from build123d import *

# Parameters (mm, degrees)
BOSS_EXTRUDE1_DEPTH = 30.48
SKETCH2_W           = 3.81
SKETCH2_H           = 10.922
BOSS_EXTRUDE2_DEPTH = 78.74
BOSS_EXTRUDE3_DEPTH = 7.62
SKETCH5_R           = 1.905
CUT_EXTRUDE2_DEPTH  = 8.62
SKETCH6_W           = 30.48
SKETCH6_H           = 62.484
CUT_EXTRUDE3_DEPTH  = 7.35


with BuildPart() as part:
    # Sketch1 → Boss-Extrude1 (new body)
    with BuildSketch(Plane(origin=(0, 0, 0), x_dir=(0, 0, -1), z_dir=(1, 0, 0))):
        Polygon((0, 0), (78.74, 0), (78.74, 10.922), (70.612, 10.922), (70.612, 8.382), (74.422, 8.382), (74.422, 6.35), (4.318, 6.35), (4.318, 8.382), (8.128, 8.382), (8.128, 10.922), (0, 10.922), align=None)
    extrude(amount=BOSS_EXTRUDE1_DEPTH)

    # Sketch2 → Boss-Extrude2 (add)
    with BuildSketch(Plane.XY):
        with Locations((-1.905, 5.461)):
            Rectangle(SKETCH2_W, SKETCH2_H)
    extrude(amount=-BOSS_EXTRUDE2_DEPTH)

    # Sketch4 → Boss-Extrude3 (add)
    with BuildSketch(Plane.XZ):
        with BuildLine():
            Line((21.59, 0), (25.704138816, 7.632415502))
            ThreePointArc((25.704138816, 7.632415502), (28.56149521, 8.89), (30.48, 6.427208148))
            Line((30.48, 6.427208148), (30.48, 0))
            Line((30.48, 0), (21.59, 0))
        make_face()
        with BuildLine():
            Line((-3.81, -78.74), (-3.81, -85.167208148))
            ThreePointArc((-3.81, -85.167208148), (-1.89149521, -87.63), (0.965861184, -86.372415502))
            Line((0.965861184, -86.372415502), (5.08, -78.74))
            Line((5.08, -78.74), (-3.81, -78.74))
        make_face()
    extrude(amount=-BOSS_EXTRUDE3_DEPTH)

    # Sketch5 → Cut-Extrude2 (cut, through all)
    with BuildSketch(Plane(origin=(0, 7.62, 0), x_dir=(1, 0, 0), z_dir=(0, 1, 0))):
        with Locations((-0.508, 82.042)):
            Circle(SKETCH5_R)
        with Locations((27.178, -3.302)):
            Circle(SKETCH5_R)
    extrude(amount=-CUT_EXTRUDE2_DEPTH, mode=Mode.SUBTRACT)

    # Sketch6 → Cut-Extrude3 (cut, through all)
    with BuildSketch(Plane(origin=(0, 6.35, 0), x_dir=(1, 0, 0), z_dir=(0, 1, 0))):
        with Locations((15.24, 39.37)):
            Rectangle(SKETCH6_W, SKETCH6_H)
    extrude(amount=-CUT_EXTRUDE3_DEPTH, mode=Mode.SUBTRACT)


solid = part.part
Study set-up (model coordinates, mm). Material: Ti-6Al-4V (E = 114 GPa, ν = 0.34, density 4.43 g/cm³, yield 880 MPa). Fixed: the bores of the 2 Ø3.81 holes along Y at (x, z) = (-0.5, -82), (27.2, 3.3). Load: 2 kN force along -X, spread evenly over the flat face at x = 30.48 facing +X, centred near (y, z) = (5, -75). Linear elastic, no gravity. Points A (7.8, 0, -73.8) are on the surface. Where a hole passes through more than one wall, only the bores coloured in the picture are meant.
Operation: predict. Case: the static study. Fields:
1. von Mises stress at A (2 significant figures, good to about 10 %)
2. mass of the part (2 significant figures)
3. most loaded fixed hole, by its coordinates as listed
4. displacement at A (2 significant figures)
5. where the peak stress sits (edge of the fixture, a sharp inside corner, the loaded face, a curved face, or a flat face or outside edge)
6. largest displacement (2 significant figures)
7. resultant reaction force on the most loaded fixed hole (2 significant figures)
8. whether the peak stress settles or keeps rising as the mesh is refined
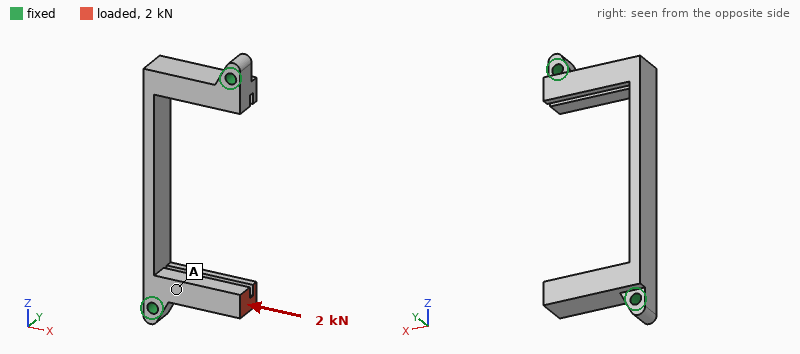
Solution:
22 MPa
39 g
(-0.5, -82)
20 µm
edge of the fixture
66 µm
2.0 kN
keeps rising
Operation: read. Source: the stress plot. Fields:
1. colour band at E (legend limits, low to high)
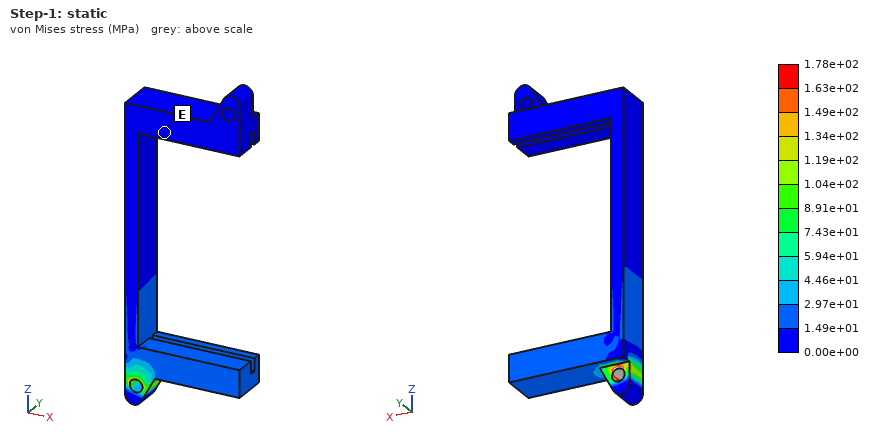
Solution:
0.00e+00 to 1.49e+01 MPa
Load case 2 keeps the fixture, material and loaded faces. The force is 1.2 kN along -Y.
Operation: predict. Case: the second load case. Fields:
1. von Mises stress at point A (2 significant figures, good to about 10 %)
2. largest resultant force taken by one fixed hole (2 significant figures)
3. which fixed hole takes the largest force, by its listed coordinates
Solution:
170 MPa
1.2 kN
(-0.5, -82)
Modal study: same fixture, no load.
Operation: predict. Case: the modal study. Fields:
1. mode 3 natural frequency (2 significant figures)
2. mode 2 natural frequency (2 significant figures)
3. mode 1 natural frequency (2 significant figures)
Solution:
5300 Hz
4000 Hz
3800 Hz
